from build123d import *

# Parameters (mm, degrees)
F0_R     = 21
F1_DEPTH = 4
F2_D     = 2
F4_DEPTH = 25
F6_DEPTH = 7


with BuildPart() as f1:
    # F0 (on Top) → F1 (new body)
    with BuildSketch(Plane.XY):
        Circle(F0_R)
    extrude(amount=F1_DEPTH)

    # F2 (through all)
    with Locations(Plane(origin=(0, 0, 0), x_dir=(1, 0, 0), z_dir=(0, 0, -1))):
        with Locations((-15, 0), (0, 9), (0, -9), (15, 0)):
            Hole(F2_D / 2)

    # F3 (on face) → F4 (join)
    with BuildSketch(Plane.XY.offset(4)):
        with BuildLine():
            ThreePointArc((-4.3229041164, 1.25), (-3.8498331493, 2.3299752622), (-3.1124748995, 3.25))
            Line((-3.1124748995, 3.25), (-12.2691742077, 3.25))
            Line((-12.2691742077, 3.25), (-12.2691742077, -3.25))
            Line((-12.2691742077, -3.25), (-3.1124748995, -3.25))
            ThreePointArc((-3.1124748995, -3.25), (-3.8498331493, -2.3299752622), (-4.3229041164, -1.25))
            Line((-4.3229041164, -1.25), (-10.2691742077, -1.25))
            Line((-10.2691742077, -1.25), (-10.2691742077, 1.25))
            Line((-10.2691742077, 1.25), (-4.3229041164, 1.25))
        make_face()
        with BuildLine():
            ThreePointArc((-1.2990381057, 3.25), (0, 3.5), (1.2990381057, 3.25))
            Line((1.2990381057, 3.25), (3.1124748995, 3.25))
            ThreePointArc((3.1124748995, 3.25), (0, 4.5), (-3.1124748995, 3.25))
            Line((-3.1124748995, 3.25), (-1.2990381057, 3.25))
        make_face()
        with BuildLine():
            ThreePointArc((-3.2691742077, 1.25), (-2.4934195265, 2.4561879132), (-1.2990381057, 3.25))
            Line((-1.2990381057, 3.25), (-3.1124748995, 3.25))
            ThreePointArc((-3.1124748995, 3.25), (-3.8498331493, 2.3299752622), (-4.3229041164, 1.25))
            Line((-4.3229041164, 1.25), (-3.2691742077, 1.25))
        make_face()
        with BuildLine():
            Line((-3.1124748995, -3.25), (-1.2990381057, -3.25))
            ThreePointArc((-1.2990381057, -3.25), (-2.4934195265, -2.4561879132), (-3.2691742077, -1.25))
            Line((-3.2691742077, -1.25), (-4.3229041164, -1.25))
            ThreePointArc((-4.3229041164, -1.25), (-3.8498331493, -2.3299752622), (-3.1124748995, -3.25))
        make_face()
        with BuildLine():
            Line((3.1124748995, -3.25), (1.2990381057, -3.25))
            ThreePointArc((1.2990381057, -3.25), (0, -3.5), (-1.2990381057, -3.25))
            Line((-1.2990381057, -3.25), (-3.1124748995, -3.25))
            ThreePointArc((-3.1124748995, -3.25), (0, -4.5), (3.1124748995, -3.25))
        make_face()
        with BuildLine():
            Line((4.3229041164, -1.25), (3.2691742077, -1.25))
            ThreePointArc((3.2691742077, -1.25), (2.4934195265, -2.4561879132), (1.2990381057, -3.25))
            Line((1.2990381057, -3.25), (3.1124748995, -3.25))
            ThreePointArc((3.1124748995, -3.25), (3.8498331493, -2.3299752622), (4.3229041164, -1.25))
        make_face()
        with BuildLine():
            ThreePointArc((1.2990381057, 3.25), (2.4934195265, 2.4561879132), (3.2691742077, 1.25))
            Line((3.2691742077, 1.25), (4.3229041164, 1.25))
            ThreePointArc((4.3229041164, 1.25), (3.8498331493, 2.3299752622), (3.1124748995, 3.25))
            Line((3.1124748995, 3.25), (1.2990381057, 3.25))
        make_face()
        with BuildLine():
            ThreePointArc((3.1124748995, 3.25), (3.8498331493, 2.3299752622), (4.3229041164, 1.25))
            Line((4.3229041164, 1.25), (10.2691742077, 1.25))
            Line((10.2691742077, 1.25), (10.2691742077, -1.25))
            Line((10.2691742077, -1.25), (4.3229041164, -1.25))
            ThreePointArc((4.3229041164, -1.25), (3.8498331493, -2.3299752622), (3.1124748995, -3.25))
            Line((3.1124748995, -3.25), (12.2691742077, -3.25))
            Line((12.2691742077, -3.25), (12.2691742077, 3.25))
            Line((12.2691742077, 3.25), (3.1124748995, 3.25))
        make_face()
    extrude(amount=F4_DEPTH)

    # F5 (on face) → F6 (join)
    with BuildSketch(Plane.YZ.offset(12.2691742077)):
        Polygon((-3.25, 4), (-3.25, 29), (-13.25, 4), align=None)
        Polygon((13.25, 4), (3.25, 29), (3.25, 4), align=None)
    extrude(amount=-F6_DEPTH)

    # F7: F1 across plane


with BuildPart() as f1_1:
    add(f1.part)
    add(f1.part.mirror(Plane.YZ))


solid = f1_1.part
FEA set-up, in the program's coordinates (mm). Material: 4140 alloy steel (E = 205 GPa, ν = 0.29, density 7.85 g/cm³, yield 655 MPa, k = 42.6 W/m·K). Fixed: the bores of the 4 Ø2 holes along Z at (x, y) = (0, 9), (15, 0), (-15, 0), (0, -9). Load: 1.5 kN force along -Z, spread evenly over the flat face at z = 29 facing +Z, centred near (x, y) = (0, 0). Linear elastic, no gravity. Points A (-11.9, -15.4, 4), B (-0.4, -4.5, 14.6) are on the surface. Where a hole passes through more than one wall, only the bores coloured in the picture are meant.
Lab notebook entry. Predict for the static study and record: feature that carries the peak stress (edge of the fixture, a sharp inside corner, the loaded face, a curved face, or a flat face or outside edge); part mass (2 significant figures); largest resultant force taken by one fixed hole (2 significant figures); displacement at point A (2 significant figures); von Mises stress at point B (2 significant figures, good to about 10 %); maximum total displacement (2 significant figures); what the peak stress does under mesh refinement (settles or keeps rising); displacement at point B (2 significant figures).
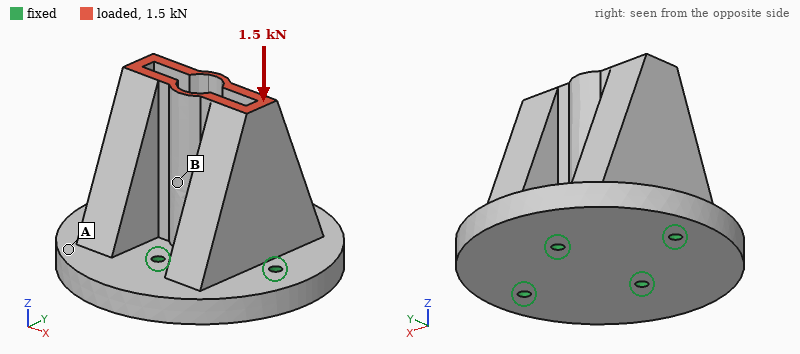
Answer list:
edge of the fixture
90 g
390 N
0.96 µm
8.6 MPa
2.3 µm
keeps rising
1.1 µm
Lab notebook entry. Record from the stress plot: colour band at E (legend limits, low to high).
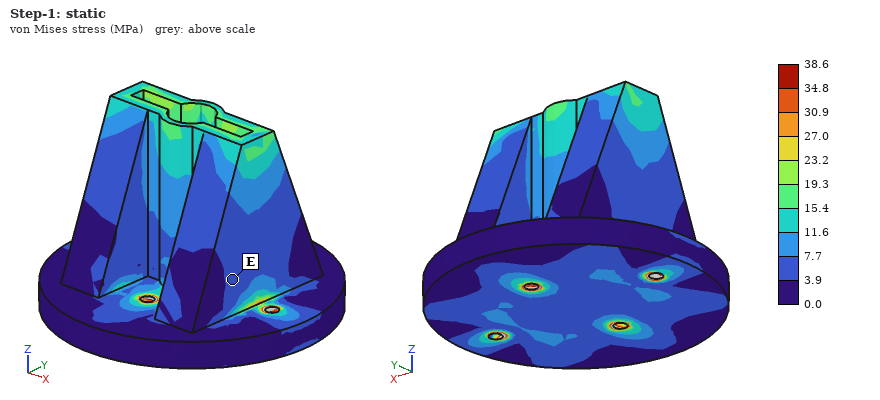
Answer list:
3.9 to 7.7 MPa
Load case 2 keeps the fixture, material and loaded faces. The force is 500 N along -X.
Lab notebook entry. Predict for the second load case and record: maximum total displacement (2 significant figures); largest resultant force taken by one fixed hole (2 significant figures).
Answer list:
5.5 µm
480 N
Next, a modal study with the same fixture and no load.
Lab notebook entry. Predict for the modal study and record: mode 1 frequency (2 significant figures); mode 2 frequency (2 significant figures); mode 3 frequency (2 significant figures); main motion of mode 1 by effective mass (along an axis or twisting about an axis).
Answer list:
11 kHz
14 kHz
14 kHz
along Y
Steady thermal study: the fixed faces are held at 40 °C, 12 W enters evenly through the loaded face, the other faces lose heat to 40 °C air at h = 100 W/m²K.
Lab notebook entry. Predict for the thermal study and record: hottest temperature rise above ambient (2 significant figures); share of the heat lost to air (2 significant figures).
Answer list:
34 K
46 %
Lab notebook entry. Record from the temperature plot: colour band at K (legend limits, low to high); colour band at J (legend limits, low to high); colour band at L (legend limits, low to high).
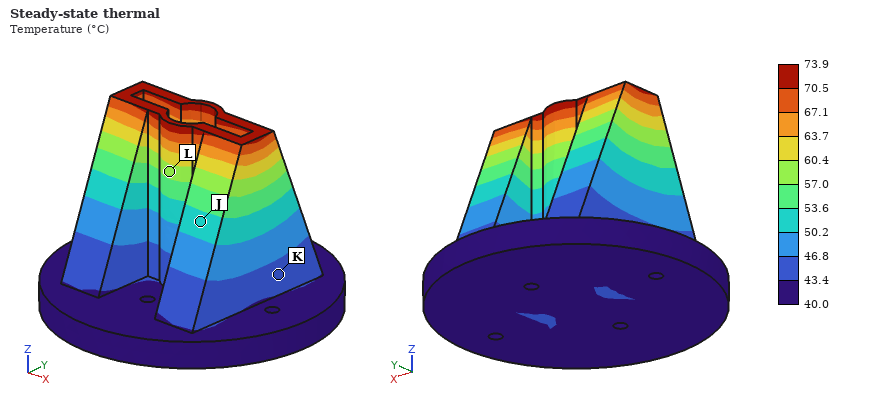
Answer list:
43.4 to 46.8 °C
50.2 to 53.6 °C
57.0 to 60.4 °C
